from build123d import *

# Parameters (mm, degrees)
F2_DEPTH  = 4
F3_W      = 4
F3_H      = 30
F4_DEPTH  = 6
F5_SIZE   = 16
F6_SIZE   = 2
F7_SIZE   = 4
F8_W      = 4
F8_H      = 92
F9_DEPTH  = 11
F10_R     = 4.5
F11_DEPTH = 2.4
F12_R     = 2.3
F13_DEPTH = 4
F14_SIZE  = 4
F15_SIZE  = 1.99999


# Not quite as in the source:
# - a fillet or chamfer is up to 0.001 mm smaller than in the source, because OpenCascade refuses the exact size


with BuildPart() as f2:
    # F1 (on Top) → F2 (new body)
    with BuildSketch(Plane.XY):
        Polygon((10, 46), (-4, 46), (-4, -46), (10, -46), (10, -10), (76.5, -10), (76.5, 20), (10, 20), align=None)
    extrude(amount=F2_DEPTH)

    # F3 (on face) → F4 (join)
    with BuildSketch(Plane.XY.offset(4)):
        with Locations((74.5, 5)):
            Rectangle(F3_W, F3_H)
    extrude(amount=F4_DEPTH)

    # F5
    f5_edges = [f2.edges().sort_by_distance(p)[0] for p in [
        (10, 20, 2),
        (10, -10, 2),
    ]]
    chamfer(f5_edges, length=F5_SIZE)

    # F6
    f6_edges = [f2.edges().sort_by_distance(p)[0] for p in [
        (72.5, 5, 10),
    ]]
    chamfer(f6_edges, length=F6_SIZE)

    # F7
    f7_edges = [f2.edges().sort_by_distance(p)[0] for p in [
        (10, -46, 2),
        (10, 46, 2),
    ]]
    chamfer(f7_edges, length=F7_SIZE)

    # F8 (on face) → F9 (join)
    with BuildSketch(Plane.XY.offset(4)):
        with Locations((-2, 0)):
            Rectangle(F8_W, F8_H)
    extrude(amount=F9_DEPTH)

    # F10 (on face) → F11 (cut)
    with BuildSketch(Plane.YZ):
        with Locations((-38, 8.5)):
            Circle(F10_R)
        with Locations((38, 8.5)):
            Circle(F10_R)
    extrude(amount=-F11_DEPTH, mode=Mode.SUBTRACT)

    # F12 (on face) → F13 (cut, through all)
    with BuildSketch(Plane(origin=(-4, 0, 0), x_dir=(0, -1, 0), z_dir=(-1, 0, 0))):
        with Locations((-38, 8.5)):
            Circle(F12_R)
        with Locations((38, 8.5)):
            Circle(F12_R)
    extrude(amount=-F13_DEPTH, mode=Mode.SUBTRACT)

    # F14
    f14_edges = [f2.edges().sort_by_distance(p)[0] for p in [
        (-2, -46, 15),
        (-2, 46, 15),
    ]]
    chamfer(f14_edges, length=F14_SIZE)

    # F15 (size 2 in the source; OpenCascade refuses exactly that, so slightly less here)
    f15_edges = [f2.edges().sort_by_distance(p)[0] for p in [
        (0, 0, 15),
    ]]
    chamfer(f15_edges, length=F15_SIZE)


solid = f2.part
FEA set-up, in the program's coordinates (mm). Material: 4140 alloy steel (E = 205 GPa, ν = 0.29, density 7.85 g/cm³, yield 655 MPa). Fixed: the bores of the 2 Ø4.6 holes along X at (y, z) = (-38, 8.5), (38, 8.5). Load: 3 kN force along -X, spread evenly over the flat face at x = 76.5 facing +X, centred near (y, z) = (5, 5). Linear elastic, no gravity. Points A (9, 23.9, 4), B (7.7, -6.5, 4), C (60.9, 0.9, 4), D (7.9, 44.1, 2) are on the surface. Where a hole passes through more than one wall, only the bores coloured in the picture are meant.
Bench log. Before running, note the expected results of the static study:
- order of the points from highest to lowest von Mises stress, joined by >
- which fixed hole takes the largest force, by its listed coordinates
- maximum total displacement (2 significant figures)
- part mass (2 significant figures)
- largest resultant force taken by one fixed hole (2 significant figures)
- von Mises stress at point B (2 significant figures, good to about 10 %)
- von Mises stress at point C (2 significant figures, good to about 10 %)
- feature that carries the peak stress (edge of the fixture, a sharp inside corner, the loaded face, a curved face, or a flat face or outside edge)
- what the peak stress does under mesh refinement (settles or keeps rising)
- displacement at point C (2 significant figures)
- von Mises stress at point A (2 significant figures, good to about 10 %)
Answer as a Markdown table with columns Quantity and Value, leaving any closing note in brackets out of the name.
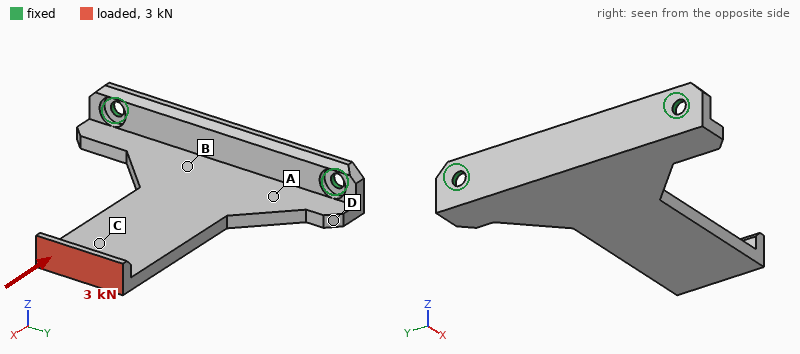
| Quantity | Value |
|---|---|
| order of the points from highest to lowest von Mises stress, joined by > | C > A > B > D |
| which fixed hole takes the largest force, by its listed coordinates | (38, 8.5) |
| maximum total displacement | 0.60 mm |
| part mass | 140 g |
| largest resultant force taken by one fixed hole | 2.0 kN |
| von Mises stress at point B | 51 MPa |
| von Mises stress at point C | 130 MPa |
| feature that carries the peak stress | edge of the fixture |
| what the peak stress does under mesh refinement | keeps rising |
| displacement at point C | 0.33 mm |
| von Mises stress at point A | 93 MPa |
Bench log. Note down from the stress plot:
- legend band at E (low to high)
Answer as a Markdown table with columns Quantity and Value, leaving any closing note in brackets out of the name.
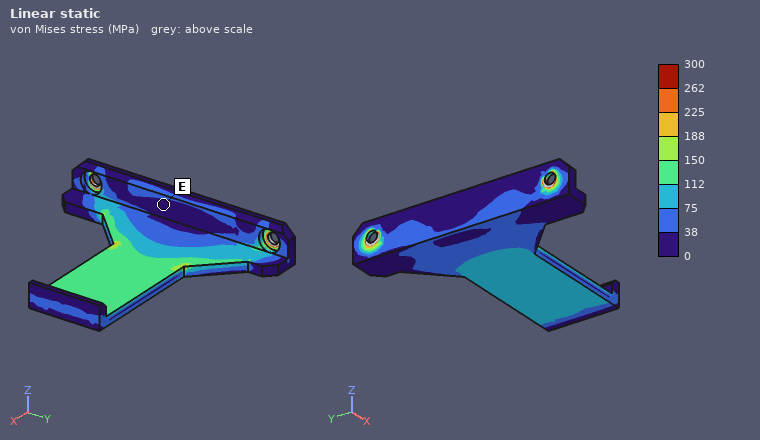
| Quantity | Value |
|---|---|
| legend band at E | 0 to 38 MPa |
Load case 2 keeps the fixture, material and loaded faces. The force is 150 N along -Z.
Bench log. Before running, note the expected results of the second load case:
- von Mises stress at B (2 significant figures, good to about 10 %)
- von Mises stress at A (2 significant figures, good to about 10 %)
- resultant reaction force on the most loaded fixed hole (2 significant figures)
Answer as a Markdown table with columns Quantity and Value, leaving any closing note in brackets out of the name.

| Quantity | Value |
|---|---|
| von Mises stress at B | 60 MPa |
| von Mises stress at A | 73 MPa |
| resultant reaction force on the most loaded fixed hole | 230 N |
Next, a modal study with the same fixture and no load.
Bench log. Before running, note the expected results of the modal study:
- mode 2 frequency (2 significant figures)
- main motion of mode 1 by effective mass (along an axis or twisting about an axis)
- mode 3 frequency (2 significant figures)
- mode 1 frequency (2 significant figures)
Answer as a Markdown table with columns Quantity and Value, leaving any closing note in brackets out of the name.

| Quantity | Value |
|---|---|
| mode 2 frequency | 2300 Hz |
| main motion of mode 1 by effective mass | along Z |
| mode 3 frequency | 2600 Hz |
| mode 1 frequency | 400 Hz |
